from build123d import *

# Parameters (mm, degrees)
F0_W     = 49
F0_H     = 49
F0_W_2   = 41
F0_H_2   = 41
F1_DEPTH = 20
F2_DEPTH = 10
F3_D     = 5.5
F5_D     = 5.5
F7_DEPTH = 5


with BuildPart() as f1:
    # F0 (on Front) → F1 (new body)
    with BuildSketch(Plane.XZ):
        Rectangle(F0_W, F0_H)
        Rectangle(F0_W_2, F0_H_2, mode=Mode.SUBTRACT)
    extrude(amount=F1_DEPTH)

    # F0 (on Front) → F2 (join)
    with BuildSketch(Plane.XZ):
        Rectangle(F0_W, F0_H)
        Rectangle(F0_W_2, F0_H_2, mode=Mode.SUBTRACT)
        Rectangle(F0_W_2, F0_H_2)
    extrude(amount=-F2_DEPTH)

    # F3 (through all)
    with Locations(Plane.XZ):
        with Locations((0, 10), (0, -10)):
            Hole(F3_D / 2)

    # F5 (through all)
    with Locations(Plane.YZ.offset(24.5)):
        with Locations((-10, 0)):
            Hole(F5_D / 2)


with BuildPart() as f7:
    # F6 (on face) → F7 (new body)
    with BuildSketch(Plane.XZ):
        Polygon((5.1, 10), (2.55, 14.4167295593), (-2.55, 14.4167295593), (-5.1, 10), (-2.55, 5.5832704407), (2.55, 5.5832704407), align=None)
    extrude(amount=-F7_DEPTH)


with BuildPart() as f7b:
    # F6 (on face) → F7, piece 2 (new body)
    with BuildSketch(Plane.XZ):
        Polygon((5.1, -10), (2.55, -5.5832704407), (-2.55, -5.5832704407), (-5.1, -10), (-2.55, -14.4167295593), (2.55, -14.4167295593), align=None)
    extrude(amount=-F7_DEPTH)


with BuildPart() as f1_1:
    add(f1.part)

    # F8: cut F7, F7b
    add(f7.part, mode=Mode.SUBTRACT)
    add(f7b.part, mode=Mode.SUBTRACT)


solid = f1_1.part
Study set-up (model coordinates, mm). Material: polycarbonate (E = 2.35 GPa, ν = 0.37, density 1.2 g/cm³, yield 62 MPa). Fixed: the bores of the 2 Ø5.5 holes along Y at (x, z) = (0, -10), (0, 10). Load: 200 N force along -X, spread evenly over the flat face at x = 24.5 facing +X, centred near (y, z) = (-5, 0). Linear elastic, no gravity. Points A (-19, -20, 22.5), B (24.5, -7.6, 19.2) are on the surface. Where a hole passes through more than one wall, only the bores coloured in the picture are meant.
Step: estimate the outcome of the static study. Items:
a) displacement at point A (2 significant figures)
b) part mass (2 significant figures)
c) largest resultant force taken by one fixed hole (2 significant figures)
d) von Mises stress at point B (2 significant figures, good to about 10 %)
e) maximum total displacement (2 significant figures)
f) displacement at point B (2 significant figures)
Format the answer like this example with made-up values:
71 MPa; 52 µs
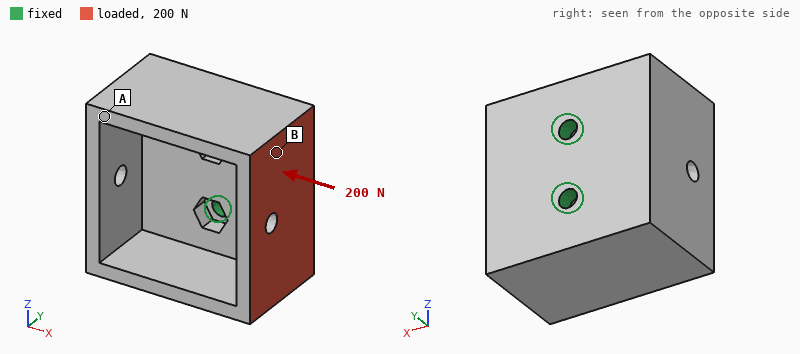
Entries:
0.16 mm; 45 g; 100 N; 2.1 MPa; 0.29 mm; 0.15 mm
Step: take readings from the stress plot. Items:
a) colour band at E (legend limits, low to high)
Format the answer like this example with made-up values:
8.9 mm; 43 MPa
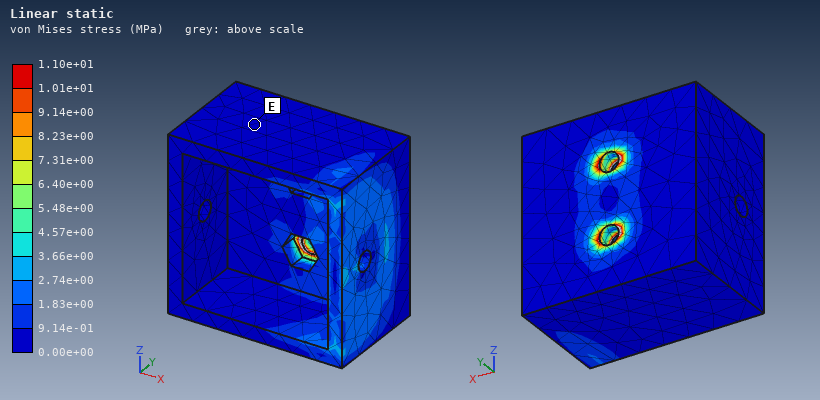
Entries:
0.00e+00 to 9.14e-01 MPa
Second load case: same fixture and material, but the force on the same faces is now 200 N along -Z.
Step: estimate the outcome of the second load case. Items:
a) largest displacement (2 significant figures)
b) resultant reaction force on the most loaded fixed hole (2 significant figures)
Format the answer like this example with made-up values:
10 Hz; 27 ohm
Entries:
0.11 mm; 250 N
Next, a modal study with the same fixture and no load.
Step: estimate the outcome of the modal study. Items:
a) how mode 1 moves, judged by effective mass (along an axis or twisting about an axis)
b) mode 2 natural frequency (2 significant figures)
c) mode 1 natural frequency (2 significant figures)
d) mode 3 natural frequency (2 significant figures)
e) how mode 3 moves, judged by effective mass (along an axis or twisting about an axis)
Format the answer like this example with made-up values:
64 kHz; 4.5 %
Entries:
along X; 1700 Hz; 890 Hz; 1800 Hz; along Z
